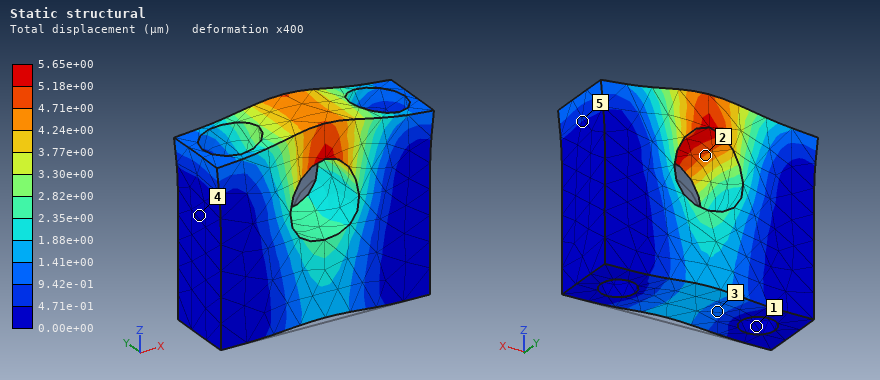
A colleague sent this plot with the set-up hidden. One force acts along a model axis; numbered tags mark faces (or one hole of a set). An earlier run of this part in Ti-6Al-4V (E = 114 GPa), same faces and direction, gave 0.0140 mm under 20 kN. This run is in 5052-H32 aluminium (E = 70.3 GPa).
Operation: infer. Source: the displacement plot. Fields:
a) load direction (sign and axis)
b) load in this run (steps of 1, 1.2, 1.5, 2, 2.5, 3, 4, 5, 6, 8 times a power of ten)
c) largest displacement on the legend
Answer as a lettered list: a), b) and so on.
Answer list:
a) +Z
b) 5 kN
c) 5.65e+00 µm
